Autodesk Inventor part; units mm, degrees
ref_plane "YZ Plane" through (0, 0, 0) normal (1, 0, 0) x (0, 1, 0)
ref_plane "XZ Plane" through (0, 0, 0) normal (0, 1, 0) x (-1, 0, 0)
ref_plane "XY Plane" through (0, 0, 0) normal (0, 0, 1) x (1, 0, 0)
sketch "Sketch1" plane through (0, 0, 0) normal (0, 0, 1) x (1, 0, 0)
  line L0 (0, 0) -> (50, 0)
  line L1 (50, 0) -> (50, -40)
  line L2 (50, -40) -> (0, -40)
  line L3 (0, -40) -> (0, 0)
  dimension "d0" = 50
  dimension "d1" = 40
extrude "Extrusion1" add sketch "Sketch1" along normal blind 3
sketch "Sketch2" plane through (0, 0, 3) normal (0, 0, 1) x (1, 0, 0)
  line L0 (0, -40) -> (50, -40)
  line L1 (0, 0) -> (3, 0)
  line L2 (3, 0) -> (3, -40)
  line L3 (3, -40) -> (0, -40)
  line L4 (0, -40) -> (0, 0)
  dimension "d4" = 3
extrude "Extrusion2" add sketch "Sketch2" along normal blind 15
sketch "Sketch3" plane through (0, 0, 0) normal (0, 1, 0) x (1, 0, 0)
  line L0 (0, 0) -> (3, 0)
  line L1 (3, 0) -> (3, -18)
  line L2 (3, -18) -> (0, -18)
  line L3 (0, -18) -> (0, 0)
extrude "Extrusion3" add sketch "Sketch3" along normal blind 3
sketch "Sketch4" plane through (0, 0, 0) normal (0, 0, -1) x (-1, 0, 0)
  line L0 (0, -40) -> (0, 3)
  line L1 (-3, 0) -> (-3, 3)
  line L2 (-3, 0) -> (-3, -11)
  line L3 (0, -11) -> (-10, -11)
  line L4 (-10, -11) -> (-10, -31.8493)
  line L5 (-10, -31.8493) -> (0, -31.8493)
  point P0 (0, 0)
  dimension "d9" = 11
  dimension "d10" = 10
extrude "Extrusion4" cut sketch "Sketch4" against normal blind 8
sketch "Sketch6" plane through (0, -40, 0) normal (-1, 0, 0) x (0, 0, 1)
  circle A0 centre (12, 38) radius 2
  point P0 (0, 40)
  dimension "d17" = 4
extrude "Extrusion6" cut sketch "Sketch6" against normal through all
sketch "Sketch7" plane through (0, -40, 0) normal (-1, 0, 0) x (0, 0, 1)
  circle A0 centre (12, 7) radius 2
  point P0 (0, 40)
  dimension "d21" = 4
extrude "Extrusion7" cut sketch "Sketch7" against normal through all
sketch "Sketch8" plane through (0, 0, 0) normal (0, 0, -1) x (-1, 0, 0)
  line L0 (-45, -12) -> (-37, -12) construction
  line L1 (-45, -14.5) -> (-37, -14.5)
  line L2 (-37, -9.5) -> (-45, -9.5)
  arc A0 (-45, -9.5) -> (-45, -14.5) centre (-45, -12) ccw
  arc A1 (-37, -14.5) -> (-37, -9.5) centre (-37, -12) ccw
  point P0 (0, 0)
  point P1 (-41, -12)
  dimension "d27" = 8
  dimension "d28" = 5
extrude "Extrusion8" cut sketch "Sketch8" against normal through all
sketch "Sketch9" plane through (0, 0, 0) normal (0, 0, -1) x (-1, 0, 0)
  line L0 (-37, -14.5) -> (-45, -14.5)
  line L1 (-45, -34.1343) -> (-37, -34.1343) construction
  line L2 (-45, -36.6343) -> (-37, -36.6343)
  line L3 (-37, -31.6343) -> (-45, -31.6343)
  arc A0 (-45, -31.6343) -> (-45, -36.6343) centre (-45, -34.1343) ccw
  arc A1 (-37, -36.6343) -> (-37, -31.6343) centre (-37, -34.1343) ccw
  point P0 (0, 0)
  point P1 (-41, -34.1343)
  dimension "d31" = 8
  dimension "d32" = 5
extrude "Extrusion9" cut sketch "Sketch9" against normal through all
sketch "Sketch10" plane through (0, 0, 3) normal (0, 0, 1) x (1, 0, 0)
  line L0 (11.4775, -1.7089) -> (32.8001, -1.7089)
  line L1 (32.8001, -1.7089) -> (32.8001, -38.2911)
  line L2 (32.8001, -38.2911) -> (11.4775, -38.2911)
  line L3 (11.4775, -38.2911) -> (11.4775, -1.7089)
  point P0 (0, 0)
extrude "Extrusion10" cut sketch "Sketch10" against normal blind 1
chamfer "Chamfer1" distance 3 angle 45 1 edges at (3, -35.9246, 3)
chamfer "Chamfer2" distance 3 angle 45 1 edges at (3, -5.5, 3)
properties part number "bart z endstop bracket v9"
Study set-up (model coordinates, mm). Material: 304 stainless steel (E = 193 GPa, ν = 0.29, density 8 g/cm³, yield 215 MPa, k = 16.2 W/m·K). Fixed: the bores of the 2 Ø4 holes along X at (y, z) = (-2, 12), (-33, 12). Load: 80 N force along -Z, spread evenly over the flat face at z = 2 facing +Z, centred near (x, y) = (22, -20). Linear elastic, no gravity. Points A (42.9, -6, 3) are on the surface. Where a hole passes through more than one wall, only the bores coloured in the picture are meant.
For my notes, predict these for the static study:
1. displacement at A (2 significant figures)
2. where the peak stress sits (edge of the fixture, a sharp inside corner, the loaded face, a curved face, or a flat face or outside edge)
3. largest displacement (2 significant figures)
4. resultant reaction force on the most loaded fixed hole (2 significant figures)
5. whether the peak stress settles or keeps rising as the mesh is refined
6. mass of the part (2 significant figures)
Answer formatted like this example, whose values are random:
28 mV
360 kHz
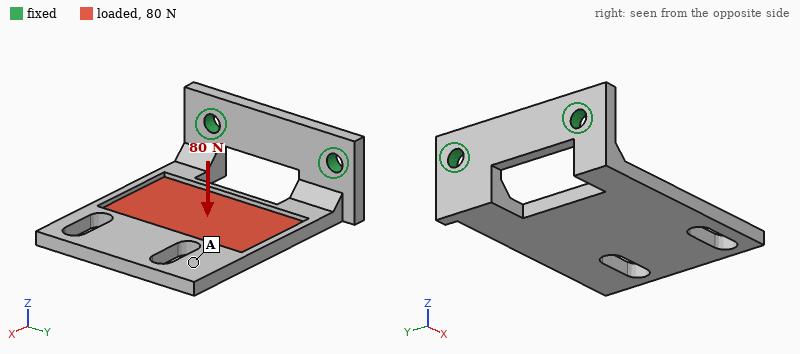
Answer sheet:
0.11 mm
edge of the fixture
0.14 mm
42 N
keeps rising
47 g
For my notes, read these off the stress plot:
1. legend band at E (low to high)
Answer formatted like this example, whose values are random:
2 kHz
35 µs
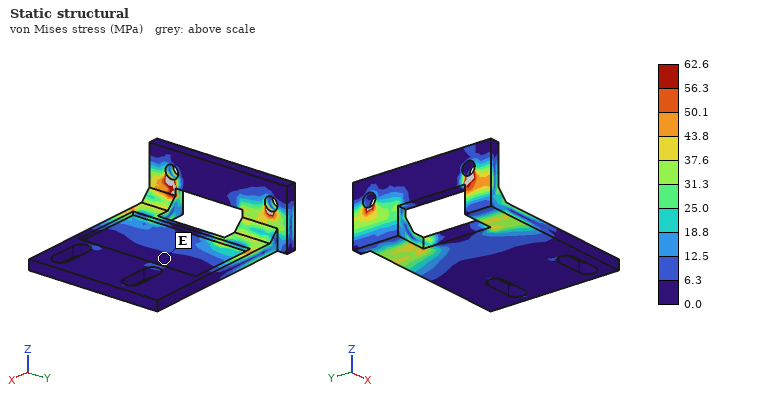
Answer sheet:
0.0 to 6.3 MPa
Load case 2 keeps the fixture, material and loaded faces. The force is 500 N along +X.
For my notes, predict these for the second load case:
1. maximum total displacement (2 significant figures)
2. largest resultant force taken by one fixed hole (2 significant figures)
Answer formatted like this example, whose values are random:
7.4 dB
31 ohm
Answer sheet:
74 µm
260 N
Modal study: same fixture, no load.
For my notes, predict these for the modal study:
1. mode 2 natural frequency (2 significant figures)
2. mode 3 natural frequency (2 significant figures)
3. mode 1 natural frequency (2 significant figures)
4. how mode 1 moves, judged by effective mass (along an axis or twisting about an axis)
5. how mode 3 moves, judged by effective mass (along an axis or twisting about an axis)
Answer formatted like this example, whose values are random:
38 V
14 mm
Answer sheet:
1900 Hz
3200 Hz
640 Hz
along Z
along Y
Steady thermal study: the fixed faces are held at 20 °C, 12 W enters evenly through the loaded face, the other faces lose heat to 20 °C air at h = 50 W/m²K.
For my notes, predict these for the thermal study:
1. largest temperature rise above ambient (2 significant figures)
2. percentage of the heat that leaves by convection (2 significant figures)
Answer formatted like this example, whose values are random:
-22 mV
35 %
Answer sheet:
85 K
79 %
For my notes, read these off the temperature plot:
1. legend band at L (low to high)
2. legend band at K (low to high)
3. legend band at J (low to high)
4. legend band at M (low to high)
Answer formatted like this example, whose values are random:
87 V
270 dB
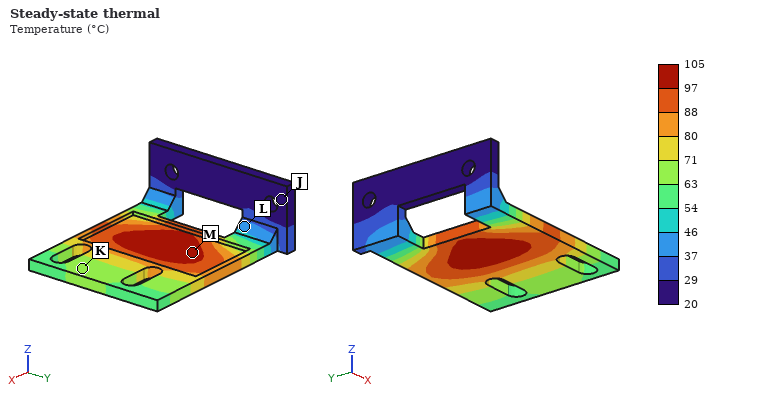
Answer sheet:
37 to 46 °C
63 to 71 °C
20 to 29 °C
97 to 105 °C
